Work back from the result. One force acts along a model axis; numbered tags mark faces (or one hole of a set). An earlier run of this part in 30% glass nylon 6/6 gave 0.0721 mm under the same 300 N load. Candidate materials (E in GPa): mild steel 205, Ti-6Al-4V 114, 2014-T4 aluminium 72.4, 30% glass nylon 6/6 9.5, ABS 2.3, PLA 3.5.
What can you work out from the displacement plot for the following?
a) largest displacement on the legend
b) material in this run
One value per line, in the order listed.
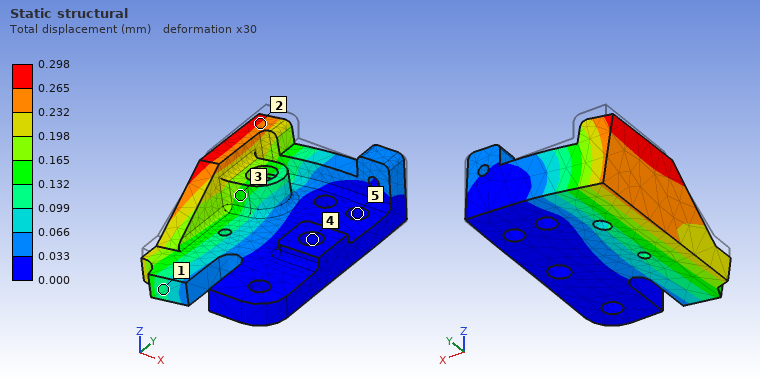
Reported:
0.298 mm
ABS
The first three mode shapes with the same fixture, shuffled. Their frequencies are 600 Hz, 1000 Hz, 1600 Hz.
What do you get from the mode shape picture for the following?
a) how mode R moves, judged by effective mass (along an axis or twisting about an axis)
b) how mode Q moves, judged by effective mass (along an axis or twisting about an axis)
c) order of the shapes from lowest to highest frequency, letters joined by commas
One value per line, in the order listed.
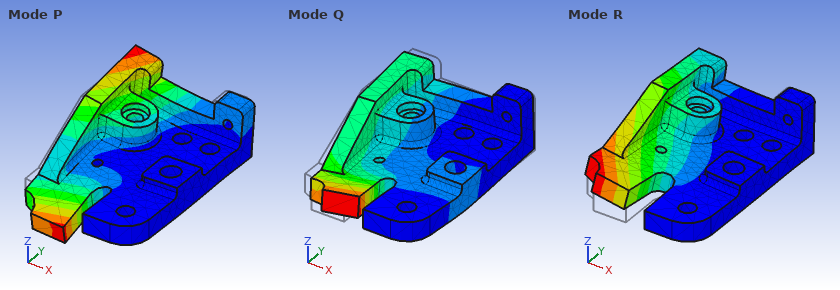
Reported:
along Z
along Y
R, P, Q
